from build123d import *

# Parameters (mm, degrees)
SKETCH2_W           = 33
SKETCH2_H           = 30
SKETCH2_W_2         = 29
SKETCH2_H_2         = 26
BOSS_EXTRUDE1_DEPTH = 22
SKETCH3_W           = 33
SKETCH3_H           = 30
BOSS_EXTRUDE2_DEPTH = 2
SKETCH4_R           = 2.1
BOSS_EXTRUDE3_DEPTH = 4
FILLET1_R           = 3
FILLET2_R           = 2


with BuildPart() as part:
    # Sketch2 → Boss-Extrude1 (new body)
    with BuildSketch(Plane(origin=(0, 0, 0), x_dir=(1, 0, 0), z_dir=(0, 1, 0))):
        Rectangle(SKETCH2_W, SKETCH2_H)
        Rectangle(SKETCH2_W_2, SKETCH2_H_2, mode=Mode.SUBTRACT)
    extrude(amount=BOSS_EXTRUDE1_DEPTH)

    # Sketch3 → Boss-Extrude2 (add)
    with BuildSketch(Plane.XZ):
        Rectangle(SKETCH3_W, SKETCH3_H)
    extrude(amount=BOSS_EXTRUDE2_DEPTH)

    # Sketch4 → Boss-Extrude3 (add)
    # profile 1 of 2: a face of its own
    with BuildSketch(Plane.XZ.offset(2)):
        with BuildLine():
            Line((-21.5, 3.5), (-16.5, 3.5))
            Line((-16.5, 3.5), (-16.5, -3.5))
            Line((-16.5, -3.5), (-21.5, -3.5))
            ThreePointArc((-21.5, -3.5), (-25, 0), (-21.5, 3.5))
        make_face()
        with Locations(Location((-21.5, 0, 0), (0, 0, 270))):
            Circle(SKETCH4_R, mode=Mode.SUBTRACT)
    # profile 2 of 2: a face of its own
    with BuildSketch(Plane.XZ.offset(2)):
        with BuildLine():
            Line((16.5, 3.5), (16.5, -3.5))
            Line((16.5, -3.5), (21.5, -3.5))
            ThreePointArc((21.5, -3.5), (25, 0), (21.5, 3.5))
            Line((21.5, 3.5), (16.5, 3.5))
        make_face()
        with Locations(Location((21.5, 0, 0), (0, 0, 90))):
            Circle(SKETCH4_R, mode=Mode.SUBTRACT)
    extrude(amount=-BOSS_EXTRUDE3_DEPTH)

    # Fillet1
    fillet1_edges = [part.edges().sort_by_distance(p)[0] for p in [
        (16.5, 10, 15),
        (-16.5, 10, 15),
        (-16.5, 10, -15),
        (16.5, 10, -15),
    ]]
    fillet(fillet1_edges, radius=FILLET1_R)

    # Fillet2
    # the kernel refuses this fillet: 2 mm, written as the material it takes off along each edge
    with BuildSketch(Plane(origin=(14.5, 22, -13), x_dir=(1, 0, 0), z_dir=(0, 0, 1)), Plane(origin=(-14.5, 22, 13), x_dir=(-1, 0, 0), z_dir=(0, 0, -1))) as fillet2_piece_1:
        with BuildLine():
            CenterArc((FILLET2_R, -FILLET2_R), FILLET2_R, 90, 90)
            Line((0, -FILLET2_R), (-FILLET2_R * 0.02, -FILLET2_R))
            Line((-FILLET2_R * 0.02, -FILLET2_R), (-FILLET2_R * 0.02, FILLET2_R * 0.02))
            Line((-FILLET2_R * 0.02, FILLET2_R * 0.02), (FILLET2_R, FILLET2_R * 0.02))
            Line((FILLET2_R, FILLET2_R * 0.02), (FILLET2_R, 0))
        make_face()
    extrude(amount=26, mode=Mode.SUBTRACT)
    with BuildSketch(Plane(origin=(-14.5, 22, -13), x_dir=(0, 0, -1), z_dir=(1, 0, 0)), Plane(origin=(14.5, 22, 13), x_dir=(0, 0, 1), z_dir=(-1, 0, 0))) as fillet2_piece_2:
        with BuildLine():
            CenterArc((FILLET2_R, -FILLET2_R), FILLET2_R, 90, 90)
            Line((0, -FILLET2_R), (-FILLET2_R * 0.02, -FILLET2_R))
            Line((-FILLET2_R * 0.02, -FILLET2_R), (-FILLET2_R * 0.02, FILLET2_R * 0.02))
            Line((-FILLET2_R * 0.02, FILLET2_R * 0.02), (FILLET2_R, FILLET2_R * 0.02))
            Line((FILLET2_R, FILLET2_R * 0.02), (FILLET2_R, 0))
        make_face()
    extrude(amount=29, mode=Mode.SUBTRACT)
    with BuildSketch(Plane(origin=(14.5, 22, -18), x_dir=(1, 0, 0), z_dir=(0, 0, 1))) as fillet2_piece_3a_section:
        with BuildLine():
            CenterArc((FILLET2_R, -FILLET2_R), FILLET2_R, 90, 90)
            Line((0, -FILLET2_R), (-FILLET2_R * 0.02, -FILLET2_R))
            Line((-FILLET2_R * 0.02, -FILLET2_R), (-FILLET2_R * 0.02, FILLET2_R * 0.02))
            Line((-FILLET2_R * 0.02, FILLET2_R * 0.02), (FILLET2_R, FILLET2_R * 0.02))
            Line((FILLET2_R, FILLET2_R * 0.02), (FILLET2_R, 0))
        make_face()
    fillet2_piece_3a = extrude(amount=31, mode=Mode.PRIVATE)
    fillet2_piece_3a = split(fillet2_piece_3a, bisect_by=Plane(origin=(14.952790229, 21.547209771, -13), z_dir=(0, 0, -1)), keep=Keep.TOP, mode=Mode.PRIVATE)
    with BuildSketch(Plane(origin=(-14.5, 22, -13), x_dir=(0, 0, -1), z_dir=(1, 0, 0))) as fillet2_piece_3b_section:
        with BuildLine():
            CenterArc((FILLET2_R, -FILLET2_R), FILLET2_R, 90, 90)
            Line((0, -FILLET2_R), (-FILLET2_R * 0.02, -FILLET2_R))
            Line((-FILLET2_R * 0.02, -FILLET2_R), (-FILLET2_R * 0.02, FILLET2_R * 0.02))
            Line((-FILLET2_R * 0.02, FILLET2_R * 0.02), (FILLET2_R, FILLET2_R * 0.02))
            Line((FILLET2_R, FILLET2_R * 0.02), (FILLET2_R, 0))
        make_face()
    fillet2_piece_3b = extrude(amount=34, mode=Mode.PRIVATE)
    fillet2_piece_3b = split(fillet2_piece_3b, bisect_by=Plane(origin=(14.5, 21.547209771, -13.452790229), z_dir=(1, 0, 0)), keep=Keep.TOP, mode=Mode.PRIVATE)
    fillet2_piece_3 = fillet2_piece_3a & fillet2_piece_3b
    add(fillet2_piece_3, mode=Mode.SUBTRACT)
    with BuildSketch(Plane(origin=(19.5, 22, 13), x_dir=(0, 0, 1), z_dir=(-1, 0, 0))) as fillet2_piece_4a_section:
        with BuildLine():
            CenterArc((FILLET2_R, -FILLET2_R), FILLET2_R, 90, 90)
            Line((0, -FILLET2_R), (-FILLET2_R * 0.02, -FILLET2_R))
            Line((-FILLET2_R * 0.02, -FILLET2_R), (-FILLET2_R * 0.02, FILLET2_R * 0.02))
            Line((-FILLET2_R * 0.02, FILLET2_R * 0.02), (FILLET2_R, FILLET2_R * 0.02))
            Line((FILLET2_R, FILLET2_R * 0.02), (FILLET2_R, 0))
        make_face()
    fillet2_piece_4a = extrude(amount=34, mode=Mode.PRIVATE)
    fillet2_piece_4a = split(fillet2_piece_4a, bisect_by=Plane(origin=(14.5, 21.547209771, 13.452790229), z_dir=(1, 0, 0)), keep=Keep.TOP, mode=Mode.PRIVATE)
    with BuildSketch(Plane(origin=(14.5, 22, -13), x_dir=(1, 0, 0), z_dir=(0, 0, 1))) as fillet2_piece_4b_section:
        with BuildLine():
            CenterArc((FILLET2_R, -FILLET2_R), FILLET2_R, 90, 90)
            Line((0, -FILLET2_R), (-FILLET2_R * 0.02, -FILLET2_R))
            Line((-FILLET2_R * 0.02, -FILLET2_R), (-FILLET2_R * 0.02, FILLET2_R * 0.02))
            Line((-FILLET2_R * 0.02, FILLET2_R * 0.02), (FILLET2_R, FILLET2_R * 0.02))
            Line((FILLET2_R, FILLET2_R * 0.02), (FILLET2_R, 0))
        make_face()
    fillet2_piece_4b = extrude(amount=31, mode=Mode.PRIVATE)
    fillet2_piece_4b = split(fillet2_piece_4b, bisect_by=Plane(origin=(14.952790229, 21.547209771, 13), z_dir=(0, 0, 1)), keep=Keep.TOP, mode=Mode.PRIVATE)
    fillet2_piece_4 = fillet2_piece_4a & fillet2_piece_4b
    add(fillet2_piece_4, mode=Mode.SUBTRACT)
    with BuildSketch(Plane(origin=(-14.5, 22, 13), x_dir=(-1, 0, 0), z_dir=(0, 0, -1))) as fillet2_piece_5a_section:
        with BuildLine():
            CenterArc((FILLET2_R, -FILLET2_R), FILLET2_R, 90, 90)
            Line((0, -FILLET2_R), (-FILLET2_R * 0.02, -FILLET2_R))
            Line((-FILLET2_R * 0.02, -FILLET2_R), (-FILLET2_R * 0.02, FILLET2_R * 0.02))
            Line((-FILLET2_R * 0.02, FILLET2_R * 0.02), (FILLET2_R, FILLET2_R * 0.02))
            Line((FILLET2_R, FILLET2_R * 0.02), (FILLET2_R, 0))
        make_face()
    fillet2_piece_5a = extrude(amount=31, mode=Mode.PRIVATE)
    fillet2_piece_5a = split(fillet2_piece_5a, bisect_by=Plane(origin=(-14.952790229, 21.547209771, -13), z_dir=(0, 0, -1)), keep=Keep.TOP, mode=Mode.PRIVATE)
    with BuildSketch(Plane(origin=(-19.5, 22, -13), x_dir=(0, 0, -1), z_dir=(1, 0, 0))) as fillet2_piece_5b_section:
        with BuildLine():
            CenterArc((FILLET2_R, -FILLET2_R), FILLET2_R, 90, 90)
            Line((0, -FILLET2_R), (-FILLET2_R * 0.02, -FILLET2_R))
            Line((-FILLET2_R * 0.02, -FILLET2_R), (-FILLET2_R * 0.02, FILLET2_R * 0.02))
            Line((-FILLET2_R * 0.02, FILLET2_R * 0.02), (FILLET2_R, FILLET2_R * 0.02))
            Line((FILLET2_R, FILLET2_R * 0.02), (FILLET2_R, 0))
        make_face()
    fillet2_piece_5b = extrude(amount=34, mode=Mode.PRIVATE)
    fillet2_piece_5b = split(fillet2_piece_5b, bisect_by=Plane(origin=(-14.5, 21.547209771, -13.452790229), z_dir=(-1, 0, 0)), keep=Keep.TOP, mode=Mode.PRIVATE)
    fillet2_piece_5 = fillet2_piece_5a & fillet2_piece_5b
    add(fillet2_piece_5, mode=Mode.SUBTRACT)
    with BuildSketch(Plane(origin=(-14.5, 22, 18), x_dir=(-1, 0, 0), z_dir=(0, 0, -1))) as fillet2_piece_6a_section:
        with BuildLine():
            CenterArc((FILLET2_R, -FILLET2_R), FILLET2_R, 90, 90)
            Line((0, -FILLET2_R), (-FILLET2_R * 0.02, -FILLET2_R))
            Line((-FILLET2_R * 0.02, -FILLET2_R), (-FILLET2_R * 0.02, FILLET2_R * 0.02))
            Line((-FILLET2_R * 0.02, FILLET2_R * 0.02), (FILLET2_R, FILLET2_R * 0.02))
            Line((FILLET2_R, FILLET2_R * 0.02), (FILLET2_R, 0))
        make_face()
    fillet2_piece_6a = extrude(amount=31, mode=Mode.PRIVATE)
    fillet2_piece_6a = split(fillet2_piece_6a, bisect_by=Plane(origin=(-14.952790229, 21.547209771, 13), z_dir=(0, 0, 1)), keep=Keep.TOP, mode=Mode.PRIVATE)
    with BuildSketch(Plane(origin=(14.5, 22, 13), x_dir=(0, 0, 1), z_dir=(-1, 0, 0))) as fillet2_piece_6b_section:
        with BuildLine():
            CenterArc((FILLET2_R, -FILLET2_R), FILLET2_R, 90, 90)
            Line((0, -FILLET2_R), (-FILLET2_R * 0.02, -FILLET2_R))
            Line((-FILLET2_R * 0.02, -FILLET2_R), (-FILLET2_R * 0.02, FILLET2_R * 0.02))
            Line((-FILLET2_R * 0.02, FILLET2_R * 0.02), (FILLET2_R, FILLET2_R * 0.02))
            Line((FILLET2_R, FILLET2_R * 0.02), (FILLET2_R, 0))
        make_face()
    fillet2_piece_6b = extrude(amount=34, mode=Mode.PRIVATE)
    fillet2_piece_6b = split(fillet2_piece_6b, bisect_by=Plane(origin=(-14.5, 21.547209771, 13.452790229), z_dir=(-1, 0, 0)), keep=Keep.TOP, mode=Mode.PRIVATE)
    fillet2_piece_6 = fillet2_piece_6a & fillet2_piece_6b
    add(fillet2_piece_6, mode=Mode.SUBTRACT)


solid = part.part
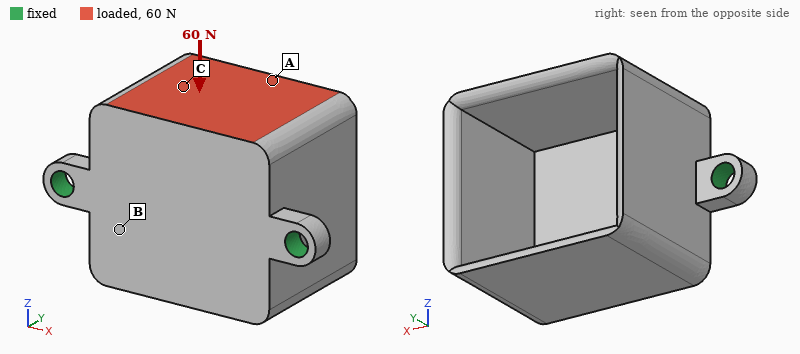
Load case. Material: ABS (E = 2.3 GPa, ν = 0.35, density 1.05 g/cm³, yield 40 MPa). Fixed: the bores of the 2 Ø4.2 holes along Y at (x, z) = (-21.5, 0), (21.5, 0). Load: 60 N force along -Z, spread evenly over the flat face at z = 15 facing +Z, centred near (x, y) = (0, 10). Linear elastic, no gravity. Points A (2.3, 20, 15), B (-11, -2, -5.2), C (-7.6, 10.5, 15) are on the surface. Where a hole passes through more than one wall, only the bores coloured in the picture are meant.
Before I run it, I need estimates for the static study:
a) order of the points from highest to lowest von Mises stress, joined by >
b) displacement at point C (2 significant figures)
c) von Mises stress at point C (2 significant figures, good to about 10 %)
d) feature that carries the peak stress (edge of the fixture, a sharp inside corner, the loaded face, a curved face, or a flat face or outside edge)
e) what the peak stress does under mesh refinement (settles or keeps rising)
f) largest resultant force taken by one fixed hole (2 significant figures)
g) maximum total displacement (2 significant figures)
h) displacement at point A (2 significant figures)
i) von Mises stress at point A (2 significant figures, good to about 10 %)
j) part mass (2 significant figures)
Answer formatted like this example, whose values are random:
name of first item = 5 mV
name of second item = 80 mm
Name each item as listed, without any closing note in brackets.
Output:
order of the points from highest to lowest von Mises stress, joined by > = A > C > B
displacement at point C = 0.37 mm
von Mises stress at point C = 4.1 MPa
feature that carries the peak stress = edge of the fixture
what the peak stress does under mesh refinement = keeps rising
largest resultant force taken by one fixed hole = 31 N
maximum total displacement = 0.71 mm
displacement at point A = 0.65 mm
von Mises stress at point A = 6.7 MPa
part mass = 7.6 g
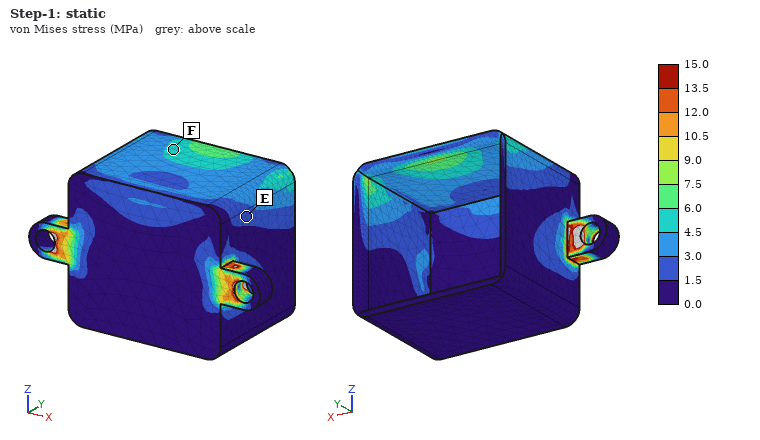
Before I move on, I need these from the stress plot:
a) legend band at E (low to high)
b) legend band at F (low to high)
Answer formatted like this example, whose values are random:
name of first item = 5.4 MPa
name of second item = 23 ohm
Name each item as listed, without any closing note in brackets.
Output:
legend band at E = 1.5 to 3.0 MPa
legend band at F = 4.5 to 6.0 MPa
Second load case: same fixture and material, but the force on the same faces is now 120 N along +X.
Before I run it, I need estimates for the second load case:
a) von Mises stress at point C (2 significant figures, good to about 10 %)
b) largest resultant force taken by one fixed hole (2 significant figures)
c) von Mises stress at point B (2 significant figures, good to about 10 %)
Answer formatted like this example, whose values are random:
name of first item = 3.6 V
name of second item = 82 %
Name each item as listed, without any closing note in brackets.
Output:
von Mises stress at point C = 1.8 MPa
largest resultant force taken by one fixed hole = 84 N
von Mises stress at point B = 1.8 MPa
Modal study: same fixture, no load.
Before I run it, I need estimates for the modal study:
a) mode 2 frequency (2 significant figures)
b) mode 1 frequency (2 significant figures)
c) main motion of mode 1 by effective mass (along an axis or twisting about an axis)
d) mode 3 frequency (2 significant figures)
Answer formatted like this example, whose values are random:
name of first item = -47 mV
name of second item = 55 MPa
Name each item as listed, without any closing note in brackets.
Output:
mode 2 frequency = 1400 Hz
mode 1 frequency = 760 Hz
main motion of mode 1 by effective mass = along Z
mode 3 frequency = 2200 Hz
